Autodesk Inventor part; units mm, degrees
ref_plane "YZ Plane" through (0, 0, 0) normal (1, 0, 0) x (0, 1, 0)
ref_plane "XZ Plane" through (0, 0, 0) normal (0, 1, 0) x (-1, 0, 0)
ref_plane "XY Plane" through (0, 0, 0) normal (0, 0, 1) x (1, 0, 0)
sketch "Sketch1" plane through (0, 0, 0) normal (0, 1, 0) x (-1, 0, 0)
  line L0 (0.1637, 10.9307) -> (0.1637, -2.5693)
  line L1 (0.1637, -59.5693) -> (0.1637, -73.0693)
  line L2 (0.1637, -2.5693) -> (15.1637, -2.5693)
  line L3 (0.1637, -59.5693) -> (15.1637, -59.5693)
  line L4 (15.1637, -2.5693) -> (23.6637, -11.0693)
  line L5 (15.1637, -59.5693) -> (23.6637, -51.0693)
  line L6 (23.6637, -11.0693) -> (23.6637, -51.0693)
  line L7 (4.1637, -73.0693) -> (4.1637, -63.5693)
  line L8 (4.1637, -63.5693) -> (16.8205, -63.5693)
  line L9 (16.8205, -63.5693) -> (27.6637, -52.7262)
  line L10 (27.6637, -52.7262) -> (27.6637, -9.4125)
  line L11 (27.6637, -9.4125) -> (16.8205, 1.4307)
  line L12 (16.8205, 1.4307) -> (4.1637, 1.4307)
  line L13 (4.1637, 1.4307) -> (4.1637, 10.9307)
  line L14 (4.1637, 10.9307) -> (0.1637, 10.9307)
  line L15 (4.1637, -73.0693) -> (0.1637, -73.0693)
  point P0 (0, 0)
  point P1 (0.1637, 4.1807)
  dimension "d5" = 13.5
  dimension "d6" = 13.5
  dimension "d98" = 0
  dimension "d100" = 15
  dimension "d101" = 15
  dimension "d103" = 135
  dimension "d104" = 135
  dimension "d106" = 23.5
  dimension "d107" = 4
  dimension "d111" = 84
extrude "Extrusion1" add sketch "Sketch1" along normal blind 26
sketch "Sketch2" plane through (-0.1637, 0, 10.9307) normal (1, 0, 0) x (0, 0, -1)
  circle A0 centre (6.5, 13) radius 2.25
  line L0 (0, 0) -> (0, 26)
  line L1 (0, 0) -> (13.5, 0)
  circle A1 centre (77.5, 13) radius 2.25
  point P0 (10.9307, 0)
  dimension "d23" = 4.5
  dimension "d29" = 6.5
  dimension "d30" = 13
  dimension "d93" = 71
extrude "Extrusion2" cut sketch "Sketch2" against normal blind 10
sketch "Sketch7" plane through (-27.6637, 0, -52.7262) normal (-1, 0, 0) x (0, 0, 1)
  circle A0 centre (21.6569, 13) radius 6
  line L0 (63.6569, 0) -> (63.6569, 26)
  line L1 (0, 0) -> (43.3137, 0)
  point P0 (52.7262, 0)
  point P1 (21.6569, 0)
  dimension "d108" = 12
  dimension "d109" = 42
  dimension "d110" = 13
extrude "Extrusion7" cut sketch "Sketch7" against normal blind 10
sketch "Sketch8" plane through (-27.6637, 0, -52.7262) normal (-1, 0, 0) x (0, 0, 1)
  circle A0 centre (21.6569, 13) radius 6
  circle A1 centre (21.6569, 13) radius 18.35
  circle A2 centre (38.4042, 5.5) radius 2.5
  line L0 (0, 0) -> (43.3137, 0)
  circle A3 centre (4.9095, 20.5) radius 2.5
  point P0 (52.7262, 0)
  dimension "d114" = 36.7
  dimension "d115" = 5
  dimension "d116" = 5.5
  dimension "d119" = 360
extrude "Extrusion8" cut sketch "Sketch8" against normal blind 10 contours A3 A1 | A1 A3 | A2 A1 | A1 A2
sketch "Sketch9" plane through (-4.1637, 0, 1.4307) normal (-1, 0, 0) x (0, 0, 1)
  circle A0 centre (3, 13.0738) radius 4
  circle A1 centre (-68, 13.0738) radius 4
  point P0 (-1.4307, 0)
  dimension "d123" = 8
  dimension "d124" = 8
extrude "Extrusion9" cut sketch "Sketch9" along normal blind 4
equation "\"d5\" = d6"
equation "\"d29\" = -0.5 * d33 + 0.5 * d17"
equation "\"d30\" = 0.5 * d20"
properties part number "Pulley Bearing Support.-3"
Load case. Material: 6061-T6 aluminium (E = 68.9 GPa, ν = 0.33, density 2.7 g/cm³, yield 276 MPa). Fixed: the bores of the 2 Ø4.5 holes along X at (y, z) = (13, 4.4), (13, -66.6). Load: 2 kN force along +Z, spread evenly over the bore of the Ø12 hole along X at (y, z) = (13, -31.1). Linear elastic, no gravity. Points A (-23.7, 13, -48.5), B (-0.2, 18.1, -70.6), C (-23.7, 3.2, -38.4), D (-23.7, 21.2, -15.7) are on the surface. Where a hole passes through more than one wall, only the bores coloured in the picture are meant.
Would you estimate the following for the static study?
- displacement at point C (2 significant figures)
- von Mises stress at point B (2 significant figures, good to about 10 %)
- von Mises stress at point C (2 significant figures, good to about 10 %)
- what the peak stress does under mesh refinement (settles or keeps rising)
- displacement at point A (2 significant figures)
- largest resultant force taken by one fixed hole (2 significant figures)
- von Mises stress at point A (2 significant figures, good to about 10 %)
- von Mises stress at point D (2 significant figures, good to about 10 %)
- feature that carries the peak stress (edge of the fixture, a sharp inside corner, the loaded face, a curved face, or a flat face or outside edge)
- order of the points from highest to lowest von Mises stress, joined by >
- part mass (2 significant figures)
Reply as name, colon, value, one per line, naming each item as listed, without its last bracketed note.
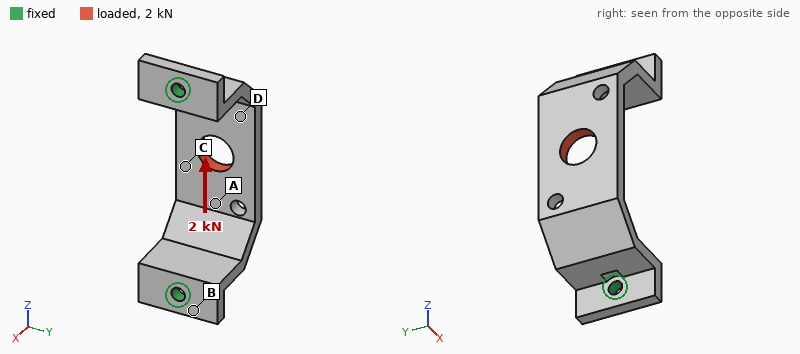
displacement at point C: 0.22 mm
von Mises stress at point B: 35 MPa
von Mises stress at point C: 63 MPa
what the peak stress does under mesh refinement: keeps rising
displacement at point A: 0.22 mm
largest resultant force taken by one fixed hole: 1.1 kN
von Mises stress at point A: 120 MPa
von Mises stress at point D: 100 MPa
feature that carries the peak stress: edge of the fixture
order of the points from highest to lowest von Mises stress, joined by >: A > D > C > B
part mass: 32 g
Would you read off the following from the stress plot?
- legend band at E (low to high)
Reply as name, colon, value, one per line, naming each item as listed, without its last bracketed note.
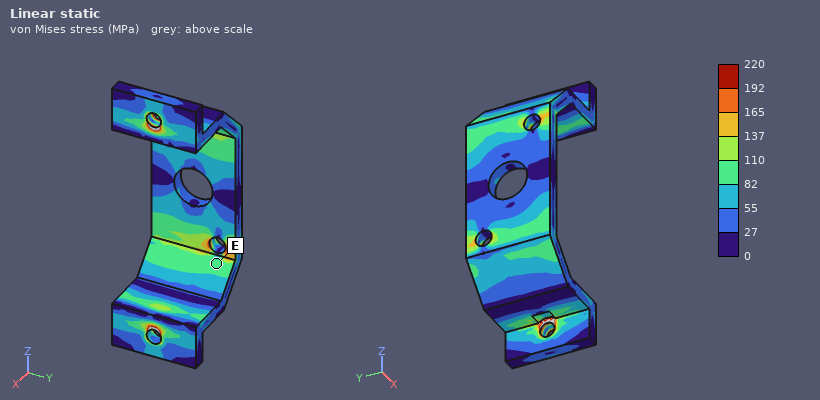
legend band at E: 82 to 110 MPa
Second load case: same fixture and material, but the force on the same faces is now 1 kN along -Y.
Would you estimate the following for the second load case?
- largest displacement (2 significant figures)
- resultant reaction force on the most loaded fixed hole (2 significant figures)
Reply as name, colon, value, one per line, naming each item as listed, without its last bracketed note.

largest displacement: 0.14 mm
resultant reaction force on the most loaded fixed hole: 500 N
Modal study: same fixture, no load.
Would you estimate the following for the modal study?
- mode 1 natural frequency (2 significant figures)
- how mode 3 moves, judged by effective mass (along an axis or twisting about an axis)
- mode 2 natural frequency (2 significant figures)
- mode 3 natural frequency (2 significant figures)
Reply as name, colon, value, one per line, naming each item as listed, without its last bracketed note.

mode 1 natural frequency: 3500 Hz
how mode 3 moves, judged by effective mass: twisting about X
mode 2 natural frequency: 3600 Hz
mode 3 natural frequency: 5700 Hz
